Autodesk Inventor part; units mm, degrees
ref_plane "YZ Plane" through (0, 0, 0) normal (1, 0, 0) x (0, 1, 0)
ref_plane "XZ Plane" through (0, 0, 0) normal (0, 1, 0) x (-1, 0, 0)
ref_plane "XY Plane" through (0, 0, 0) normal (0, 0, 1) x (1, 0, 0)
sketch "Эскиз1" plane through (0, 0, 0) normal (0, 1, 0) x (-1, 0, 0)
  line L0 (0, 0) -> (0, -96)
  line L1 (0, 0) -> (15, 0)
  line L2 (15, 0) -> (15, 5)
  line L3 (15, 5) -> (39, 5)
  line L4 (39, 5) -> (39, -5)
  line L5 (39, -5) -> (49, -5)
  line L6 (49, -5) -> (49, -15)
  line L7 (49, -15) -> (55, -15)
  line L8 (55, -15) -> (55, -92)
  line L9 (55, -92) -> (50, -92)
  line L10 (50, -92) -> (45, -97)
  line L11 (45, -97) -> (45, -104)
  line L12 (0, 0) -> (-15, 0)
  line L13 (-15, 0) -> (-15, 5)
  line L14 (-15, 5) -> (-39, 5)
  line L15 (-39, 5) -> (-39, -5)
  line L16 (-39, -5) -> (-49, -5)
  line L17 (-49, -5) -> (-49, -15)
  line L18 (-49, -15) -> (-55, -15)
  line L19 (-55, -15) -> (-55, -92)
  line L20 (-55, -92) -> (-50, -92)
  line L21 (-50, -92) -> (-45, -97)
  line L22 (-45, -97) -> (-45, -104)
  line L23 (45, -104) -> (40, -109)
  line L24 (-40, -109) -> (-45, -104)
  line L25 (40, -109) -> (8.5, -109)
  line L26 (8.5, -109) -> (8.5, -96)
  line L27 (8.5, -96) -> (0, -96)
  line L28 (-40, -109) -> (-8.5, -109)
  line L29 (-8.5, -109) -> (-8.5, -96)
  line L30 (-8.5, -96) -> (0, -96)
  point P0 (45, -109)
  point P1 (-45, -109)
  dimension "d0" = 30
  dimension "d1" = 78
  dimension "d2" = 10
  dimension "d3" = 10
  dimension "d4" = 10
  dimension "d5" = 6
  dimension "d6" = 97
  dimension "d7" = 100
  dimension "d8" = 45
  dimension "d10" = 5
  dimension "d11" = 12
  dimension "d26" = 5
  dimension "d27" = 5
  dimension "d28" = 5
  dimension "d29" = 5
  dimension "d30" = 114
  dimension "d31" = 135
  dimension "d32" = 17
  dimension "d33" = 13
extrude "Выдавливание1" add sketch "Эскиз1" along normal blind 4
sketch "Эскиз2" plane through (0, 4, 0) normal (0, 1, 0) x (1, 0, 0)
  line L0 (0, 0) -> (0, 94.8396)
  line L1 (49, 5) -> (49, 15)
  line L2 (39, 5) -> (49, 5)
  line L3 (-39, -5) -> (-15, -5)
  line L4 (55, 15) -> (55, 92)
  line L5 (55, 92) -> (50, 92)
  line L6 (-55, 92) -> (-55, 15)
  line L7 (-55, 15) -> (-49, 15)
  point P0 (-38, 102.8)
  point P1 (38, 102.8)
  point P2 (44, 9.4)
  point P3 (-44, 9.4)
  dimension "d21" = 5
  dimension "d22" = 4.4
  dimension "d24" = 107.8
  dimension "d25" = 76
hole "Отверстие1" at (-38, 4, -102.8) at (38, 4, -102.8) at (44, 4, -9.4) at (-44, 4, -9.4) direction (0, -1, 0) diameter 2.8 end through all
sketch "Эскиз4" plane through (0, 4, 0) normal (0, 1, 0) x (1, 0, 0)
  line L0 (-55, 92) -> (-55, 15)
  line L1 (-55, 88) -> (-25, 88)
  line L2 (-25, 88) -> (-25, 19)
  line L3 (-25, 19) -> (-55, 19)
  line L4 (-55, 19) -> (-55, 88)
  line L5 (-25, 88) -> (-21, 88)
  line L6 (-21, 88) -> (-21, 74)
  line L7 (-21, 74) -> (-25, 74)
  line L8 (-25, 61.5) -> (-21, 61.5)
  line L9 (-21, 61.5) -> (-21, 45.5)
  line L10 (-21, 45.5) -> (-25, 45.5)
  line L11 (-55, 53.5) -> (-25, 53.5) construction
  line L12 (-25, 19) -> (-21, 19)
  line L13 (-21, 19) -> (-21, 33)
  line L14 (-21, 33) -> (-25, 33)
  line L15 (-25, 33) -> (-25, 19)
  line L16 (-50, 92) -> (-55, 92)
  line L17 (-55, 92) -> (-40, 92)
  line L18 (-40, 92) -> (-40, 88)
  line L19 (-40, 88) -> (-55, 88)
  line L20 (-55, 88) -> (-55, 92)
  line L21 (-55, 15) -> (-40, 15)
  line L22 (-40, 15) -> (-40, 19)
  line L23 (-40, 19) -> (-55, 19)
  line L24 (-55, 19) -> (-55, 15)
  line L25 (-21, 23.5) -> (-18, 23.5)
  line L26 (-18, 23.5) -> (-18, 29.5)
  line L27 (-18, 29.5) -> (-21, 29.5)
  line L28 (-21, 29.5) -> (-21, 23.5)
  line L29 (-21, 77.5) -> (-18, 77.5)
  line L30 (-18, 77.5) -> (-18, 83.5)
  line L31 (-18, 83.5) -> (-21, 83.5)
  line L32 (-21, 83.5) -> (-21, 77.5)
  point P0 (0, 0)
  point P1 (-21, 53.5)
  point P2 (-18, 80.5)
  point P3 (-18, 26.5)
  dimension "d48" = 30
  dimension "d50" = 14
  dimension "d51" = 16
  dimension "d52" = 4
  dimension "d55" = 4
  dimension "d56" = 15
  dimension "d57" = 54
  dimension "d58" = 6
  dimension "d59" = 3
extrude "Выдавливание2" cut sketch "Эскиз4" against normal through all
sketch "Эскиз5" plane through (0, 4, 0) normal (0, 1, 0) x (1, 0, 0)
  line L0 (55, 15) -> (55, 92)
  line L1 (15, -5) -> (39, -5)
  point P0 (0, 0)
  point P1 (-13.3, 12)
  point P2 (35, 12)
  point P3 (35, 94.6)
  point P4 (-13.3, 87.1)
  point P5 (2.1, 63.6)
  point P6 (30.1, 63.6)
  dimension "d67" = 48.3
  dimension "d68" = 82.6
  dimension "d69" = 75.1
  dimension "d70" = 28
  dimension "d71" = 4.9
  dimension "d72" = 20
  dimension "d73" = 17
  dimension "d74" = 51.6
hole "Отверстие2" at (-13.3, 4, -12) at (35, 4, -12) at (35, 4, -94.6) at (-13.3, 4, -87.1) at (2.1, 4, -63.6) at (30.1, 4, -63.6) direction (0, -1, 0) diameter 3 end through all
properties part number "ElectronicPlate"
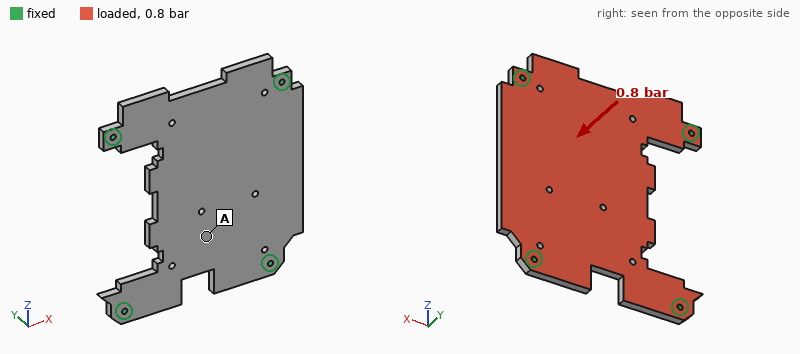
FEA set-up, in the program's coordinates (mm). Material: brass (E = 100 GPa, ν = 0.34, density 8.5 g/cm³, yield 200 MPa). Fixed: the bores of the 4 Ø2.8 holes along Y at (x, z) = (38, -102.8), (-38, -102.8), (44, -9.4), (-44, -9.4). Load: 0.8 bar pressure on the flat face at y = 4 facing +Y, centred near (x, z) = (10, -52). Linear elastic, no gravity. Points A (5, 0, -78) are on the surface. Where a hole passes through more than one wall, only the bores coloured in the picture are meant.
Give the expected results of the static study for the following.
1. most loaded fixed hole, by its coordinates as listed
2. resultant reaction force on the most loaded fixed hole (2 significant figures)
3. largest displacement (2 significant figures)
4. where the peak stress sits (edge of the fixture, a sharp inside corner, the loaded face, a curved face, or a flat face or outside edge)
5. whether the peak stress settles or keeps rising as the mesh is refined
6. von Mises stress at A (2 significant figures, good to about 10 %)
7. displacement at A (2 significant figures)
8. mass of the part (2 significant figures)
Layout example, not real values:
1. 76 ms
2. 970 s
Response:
1. (44, -9.4)
2. 240 N
3. 99 µm
4. edge of the fixture
5. keeps rising
6. 9.7 MPa
7. 65 µm
8. 300 g
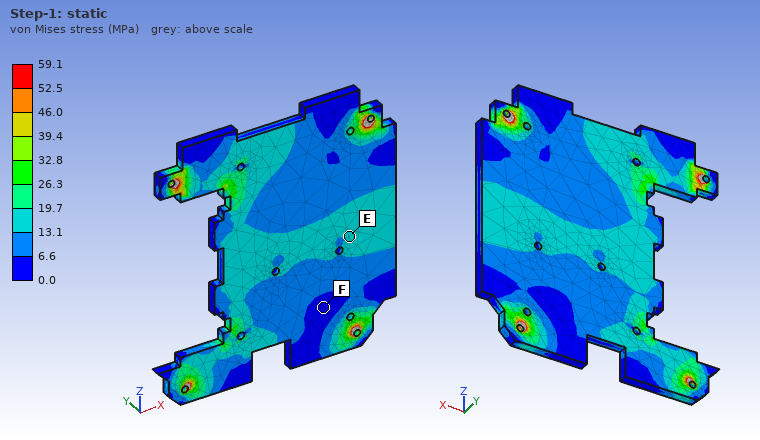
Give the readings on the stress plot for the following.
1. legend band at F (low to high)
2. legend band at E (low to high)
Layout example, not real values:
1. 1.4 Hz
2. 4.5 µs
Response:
1. 0.0 to 6.6 MPa
2. 13.1 to 19.7 MPa
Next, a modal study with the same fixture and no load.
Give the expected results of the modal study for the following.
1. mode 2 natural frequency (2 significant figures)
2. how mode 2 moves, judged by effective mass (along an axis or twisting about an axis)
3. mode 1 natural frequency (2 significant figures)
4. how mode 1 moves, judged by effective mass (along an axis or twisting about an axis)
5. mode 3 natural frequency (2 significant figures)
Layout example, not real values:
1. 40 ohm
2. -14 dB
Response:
1. 1500 Hz
2. twisting about Z
3. 970 Hz
4. along Y
5. 1800 Hz
